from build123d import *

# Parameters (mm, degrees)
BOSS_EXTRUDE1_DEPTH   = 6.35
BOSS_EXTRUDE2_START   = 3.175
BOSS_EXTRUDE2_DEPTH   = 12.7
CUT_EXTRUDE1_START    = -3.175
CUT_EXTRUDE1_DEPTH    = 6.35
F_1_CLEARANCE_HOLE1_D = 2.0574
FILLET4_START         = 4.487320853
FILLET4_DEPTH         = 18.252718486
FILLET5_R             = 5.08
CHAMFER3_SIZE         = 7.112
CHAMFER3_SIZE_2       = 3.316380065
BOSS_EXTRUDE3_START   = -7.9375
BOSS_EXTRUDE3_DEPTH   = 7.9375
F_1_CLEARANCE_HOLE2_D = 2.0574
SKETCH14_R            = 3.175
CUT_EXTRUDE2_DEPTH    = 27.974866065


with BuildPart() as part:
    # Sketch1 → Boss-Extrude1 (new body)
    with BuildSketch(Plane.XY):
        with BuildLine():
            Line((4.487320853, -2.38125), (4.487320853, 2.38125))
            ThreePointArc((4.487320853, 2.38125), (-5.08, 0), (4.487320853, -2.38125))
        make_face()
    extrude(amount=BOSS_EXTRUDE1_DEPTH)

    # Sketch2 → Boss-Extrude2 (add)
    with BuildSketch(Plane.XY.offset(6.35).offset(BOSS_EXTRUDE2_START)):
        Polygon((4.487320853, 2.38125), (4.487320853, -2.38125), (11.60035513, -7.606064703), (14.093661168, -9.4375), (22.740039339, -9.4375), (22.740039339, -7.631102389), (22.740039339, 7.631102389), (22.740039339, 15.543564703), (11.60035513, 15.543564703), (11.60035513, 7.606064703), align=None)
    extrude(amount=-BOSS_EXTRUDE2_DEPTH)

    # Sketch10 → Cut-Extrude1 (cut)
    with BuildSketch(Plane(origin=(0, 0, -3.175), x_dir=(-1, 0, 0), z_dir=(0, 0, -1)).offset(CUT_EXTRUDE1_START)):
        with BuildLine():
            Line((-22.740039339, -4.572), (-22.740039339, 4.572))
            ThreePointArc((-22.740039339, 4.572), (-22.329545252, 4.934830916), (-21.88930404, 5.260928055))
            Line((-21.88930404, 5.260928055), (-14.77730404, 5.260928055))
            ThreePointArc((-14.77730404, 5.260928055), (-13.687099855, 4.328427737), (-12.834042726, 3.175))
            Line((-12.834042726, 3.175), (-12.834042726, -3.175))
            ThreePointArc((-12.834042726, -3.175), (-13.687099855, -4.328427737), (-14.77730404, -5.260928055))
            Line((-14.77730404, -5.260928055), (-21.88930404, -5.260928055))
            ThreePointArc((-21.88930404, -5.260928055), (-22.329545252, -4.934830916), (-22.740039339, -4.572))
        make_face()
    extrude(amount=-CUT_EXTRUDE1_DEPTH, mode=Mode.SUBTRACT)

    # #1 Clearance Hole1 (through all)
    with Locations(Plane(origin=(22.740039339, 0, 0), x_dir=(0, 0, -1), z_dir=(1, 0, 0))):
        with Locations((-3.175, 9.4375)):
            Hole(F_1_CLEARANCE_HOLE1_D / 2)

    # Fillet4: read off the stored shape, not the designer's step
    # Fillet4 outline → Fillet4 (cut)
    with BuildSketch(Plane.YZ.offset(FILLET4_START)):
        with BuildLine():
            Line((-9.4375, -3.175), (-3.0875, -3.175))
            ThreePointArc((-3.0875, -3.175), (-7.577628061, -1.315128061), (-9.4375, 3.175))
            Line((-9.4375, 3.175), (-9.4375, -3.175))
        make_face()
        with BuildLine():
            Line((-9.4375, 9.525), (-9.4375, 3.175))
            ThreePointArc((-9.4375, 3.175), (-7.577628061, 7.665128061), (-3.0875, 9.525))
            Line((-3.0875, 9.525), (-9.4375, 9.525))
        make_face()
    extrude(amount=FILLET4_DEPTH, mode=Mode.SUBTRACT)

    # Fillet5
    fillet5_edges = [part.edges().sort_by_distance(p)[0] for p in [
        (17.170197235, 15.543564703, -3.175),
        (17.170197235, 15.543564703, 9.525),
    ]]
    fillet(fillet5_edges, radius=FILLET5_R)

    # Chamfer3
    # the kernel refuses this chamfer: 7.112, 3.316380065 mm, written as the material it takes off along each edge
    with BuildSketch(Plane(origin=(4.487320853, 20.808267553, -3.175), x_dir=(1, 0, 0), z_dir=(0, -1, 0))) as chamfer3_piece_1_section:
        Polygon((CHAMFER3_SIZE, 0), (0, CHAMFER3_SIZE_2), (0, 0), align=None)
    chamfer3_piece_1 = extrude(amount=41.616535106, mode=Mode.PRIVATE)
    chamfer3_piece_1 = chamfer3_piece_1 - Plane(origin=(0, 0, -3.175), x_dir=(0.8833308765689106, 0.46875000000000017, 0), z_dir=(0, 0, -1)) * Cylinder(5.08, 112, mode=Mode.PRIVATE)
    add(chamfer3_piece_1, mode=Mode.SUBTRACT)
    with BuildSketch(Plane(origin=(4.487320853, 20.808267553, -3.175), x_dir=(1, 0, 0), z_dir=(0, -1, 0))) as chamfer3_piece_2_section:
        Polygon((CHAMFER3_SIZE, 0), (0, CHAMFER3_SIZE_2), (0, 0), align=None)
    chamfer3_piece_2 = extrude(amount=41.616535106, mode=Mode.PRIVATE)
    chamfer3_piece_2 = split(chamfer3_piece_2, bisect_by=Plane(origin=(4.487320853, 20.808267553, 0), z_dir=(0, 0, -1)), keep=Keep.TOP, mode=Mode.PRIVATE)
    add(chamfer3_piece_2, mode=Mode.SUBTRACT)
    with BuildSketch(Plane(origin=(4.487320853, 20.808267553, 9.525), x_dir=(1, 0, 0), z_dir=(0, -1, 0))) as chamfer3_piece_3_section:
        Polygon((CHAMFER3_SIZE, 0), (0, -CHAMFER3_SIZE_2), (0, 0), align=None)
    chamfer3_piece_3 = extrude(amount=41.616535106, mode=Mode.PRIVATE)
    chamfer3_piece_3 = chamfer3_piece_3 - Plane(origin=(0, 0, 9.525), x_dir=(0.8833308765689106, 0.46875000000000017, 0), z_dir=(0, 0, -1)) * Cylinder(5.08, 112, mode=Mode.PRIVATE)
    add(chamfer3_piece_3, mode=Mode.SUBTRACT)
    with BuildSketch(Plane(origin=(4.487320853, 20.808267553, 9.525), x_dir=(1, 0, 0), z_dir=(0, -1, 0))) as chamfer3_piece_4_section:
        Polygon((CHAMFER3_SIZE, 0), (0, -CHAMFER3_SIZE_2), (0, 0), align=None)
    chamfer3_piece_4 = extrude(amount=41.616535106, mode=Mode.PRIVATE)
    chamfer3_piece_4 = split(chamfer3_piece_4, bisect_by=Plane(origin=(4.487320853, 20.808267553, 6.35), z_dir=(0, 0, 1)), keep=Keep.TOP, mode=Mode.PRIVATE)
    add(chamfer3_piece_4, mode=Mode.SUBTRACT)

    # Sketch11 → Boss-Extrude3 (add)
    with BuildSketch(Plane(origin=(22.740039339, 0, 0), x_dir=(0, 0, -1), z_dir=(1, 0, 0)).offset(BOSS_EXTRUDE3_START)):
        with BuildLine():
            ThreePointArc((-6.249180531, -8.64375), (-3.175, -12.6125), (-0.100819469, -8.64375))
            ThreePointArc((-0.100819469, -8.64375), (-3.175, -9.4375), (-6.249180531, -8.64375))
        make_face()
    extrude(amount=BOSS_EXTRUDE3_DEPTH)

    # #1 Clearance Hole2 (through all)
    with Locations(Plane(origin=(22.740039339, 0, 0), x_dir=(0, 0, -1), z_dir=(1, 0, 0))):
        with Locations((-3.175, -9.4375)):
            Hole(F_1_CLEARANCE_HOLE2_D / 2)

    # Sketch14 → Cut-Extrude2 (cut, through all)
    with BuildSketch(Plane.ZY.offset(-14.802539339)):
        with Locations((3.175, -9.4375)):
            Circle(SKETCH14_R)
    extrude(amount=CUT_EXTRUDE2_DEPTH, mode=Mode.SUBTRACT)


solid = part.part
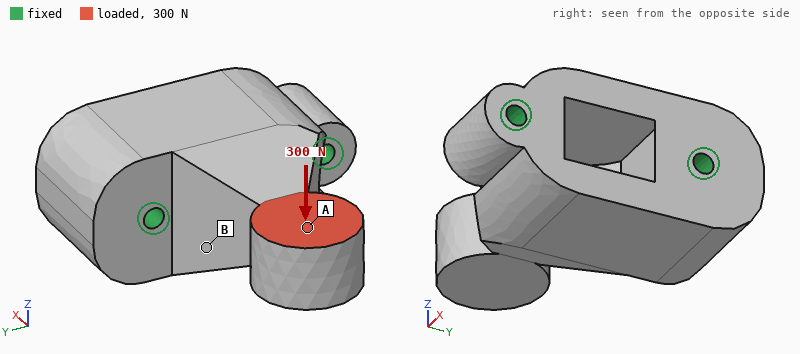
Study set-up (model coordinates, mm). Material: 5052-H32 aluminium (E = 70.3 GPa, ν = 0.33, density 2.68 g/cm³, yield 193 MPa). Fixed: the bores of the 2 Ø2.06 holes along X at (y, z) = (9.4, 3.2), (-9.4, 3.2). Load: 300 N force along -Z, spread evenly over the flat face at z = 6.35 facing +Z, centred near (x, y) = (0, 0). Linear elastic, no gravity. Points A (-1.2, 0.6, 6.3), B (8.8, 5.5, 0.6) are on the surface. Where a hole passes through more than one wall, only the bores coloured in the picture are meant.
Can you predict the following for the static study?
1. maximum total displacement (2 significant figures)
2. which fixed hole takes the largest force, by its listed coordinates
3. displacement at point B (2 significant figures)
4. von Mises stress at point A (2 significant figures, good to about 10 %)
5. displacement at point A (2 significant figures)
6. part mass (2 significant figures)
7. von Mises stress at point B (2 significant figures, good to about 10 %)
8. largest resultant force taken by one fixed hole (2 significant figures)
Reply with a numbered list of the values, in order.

1. 26 µm
2. (9.4, 3.2)
3. 4.4 µm
4. 5.8 MPa
5. 20 µm
6. 10 g
7. 14 MPa
8. 190 N
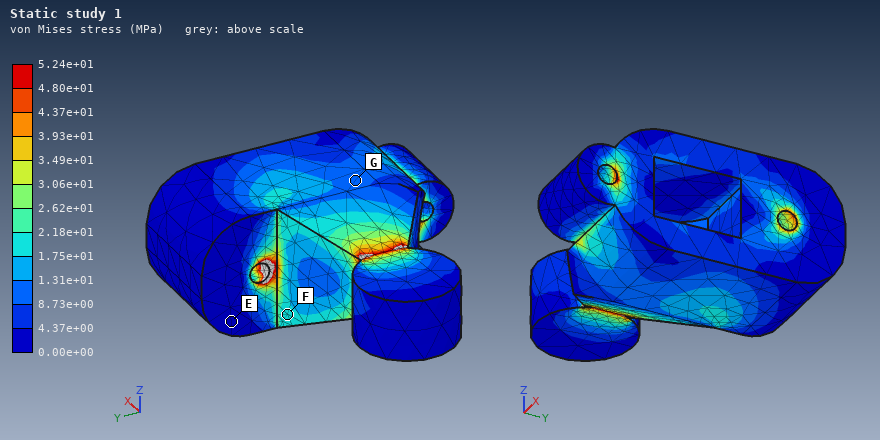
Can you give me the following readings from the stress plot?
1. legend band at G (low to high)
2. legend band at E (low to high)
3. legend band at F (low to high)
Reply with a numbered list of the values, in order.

1. 8.73e+00 to 1.31e+01 MPa
2. 0.00e+00 to 4.37e+00 MPa
3. 1.75e+01 to 2.18e+01 MPa
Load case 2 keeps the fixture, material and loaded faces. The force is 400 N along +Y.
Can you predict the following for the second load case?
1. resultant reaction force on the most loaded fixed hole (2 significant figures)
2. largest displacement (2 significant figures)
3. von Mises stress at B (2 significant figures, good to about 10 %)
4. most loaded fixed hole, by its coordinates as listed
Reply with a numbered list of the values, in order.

1. 460 N
2. 29 µm
3. 19 MPa
4. (9.4, 3.2)
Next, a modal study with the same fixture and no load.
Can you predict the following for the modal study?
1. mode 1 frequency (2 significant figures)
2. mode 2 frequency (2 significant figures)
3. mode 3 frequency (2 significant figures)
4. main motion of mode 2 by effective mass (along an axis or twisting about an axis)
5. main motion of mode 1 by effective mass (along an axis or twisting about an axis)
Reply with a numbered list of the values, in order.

1. 16 kHz
2. 20 kHz
3. 41 kHz
4. along Y
5. along Z
